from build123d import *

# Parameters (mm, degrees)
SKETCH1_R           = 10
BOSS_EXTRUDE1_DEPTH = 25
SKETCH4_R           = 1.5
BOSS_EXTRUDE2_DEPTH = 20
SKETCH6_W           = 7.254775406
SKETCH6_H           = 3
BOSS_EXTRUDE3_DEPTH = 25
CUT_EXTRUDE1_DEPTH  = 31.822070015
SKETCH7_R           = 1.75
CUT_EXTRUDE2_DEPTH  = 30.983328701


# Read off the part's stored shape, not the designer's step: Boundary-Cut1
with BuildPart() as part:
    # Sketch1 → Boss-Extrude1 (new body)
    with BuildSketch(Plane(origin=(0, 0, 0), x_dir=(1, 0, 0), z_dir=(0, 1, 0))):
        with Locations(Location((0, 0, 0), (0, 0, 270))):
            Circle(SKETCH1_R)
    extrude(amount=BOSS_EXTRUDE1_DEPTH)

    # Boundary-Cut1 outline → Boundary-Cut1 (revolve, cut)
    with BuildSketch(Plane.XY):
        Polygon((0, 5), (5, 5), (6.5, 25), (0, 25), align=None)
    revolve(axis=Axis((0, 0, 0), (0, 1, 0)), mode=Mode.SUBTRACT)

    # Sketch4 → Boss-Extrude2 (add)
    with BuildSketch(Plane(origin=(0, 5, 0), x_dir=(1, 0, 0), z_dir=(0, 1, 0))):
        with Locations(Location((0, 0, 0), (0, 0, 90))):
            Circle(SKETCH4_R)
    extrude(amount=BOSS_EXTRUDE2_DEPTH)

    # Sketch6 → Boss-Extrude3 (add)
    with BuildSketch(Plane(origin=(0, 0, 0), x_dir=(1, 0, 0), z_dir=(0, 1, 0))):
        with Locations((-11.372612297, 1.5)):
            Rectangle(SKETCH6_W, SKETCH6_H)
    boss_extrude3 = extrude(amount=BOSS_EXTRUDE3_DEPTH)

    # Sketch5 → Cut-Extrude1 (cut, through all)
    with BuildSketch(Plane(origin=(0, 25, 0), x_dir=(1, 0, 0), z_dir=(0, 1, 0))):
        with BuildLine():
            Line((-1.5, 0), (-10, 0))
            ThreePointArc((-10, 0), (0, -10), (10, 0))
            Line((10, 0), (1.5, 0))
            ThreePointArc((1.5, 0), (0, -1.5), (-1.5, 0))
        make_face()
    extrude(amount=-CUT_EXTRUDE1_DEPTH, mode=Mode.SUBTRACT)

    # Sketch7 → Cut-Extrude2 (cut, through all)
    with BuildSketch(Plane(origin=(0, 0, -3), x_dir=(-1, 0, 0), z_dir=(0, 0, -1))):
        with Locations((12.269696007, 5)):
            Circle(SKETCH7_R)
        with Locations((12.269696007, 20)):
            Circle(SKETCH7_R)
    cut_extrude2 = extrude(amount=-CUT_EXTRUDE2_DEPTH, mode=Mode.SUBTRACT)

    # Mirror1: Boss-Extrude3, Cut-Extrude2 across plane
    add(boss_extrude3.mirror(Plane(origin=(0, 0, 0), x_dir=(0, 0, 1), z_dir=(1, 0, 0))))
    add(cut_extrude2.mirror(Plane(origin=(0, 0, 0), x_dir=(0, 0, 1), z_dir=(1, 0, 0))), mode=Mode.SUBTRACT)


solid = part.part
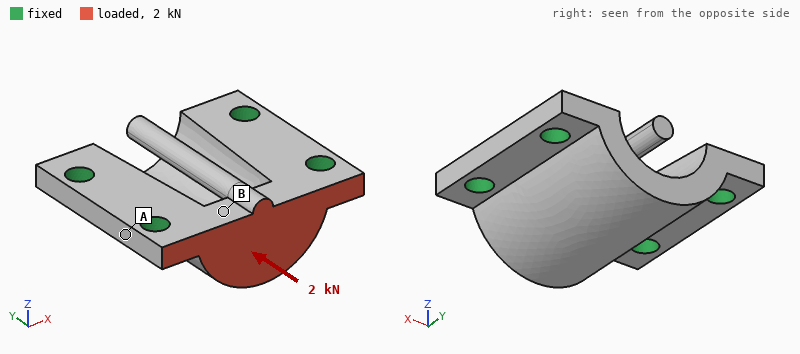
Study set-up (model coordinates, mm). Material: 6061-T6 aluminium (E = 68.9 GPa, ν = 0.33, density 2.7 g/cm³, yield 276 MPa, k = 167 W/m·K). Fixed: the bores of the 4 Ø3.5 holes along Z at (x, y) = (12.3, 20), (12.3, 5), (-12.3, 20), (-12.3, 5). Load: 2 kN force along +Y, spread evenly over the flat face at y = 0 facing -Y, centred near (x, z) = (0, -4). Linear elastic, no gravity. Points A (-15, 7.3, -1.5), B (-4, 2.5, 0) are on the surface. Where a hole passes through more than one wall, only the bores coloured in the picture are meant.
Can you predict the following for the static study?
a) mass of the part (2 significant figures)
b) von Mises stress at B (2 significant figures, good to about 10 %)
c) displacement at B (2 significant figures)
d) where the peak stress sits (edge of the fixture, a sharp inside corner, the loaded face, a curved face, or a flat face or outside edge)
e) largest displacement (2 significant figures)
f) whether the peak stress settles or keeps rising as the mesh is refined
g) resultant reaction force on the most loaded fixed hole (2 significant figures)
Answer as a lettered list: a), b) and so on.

a) 10.0 g
b) 24 MPa
c) 5.2 µm
d) edge of the fixture
e) 10 µm
f) keeps rising
g) 670 N
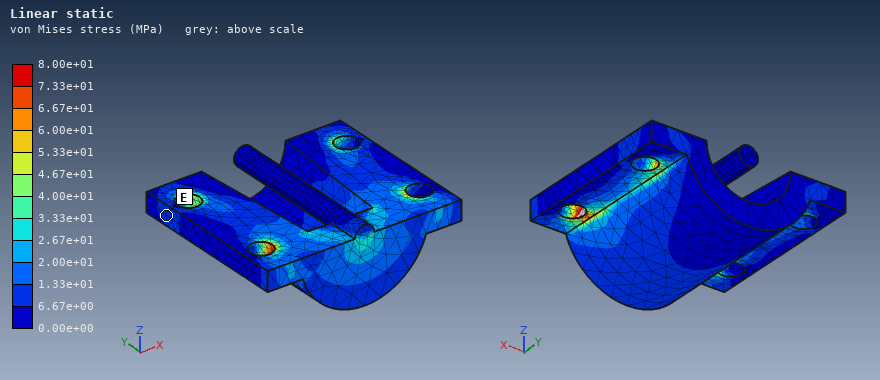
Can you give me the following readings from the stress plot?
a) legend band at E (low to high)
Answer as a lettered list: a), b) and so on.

a) 6.67e+00 to 1.33e+01 MPa
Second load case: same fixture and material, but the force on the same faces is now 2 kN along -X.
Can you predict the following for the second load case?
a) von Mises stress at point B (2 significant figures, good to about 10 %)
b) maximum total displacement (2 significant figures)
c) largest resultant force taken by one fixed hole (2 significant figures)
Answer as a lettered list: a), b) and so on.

a) 28 MPa
b) 6.4 µm
c) 980 N
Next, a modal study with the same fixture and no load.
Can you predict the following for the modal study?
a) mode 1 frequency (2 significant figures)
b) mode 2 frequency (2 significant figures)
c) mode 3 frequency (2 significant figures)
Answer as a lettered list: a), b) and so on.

a) 4600 Hz
b) 4700 Hz
c) 26 kHz
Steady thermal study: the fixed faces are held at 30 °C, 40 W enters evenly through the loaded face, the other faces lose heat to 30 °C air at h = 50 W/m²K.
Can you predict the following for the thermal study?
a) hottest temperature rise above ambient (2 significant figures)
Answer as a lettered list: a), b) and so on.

a) 20 K
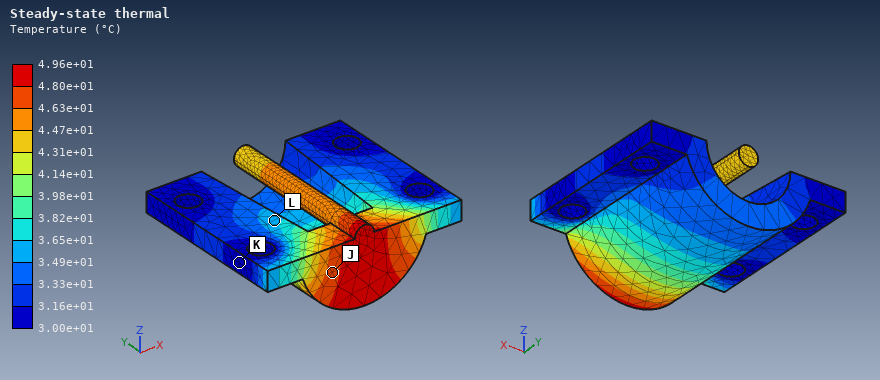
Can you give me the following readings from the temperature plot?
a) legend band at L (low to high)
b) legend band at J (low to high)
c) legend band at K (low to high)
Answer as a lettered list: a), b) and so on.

a) 3.49e+01 to 3.65e+01 °C
b) 4.63e+01 to 4.80e+01 °C
c) 3.00e+01 to 3.16e+01 °C
